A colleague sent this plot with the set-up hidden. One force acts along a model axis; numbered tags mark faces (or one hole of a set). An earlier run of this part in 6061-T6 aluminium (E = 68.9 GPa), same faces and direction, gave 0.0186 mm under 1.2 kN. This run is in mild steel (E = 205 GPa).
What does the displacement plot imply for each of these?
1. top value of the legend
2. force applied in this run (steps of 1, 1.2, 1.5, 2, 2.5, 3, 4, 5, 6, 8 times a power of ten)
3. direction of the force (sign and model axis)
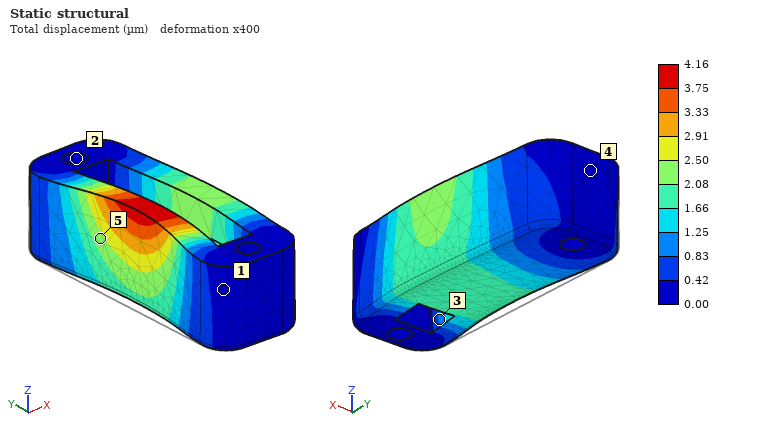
4.16 µm
800 N
+X
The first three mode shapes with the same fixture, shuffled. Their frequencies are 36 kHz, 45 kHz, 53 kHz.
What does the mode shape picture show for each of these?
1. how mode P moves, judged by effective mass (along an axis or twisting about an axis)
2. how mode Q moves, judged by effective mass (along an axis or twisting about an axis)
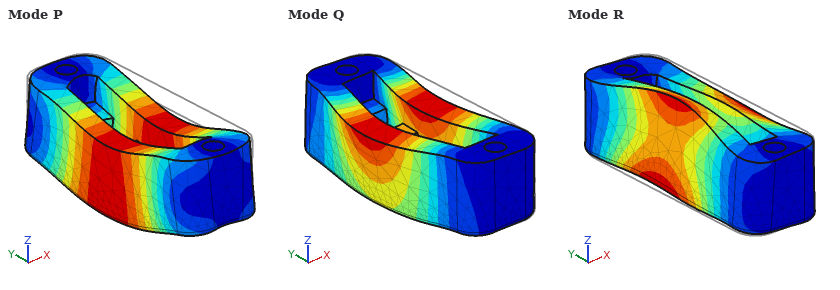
along Z
along X
